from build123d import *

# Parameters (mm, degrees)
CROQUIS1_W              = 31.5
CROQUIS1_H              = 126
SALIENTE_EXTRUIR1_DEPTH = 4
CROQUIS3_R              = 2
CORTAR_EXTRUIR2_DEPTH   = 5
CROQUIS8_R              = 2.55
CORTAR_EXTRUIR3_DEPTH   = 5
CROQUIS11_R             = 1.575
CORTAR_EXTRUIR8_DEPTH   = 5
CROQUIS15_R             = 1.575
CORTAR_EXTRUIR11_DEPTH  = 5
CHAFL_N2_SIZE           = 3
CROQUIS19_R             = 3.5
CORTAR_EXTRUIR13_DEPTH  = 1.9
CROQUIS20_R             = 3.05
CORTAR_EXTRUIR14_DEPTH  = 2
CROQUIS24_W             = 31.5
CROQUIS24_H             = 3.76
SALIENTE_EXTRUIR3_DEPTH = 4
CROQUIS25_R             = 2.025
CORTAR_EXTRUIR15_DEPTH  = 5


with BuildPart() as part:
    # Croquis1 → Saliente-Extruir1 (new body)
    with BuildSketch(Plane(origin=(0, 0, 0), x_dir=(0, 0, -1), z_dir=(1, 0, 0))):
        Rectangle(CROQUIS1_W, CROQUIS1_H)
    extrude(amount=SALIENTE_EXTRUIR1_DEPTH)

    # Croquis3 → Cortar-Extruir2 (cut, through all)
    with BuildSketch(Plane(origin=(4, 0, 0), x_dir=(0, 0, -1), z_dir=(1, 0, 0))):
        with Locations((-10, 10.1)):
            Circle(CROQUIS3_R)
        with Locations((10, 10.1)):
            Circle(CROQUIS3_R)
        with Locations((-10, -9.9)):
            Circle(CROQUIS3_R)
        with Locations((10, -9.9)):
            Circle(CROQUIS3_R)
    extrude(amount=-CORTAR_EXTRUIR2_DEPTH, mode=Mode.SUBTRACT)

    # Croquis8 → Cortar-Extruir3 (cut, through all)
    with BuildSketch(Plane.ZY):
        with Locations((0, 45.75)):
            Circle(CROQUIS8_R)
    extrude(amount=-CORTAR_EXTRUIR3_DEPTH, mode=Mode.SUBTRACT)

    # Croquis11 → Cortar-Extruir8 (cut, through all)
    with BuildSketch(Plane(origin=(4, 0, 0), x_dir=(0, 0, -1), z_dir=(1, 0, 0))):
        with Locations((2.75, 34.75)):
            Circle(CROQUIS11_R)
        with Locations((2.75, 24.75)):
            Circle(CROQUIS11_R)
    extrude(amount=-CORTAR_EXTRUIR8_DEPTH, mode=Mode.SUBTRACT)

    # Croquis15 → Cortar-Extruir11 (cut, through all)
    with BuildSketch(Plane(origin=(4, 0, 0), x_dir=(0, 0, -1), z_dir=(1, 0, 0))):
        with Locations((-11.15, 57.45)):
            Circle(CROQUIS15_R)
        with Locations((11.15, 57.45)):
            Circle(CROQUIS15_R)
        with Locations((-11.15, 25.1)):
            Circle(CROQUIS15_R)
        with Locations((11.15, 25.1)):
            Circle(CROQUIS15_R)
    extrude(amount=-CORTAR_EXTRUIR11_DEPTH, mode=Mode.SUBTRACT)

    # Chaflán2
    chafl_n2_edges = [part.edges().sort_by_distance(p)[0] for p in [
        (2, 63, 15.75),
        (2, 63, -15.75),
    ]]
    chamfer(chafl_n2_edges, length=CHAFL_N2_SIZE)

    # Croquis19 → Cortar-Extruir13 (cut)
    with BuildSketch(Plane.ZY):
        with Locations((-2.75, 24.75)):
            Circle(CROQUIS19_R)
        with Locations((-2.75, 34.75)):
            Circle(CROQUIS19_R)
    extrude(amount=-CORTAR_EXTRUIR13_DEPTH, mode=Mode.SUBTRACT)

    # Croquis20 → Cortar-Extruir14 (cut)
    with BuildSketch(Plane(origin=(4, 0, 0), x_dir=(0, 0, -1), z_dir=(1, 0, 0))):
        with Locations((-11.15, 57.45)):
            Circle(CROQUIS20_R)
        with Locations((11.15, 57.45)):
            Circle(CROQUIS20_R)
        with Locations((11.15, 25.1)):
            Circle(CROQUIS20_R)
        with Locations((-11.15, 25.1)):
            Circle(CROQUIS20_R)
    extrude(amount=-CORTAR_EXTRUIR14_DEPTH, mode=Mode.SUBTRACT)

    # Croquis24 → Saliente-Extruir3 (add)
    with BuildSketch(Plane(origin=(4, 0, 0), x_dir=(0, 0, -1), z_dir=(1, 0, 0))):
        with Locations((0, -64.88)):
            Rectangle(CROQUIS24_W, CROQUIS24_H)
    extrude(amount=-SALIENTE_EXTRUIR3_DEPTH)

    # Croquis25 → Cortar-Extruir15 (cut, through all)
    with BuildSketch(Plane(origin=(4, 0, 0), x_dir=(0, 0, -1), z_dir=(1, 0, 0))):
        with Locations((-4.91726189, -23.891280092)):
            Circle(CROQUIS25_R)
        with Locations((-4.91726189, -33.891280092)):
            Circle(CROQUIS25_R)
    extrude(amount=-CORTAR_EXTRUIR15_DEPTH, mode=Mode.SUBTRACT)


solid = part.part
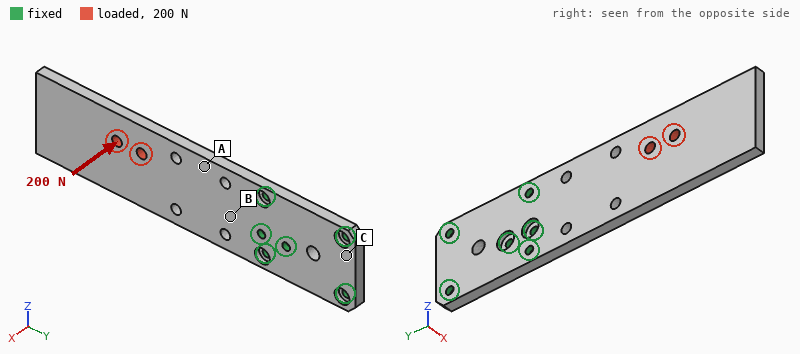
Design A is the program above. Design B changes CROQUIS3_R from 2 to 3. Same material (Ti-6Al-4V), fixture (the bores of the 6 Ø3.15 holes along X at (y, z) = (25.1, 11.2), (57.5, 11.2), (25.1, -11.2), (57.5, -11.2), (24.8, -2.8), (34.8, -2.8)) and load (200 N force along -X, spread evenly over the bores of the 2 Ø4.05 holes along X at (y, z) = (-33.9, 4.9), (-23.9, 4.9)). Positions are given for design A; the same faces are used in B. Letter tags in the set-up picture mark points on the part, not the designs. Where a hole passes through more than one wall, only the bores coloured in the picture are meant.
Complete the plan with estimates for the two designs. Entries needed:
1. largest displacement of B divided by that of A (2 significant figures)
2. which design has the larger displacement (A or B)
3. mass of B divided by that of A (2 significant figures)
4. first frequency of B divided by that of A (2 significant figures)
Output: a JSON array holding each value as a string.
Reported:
["1.1", "B", "0.98", "0.96"]
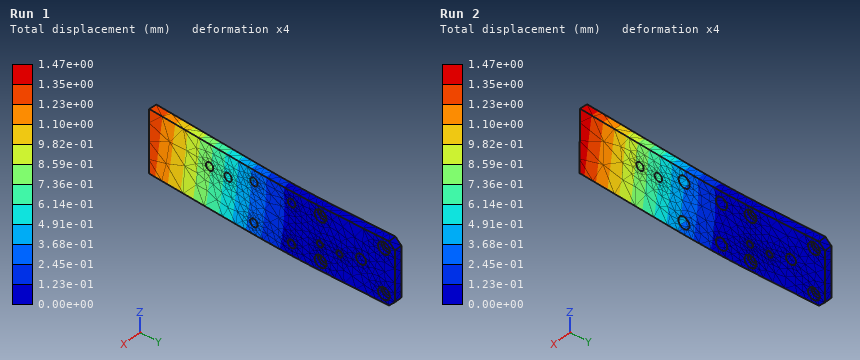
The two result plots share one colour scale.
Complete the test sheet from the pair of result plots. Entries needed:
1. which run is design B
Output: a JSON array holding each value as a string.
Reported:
["Run 2"]
